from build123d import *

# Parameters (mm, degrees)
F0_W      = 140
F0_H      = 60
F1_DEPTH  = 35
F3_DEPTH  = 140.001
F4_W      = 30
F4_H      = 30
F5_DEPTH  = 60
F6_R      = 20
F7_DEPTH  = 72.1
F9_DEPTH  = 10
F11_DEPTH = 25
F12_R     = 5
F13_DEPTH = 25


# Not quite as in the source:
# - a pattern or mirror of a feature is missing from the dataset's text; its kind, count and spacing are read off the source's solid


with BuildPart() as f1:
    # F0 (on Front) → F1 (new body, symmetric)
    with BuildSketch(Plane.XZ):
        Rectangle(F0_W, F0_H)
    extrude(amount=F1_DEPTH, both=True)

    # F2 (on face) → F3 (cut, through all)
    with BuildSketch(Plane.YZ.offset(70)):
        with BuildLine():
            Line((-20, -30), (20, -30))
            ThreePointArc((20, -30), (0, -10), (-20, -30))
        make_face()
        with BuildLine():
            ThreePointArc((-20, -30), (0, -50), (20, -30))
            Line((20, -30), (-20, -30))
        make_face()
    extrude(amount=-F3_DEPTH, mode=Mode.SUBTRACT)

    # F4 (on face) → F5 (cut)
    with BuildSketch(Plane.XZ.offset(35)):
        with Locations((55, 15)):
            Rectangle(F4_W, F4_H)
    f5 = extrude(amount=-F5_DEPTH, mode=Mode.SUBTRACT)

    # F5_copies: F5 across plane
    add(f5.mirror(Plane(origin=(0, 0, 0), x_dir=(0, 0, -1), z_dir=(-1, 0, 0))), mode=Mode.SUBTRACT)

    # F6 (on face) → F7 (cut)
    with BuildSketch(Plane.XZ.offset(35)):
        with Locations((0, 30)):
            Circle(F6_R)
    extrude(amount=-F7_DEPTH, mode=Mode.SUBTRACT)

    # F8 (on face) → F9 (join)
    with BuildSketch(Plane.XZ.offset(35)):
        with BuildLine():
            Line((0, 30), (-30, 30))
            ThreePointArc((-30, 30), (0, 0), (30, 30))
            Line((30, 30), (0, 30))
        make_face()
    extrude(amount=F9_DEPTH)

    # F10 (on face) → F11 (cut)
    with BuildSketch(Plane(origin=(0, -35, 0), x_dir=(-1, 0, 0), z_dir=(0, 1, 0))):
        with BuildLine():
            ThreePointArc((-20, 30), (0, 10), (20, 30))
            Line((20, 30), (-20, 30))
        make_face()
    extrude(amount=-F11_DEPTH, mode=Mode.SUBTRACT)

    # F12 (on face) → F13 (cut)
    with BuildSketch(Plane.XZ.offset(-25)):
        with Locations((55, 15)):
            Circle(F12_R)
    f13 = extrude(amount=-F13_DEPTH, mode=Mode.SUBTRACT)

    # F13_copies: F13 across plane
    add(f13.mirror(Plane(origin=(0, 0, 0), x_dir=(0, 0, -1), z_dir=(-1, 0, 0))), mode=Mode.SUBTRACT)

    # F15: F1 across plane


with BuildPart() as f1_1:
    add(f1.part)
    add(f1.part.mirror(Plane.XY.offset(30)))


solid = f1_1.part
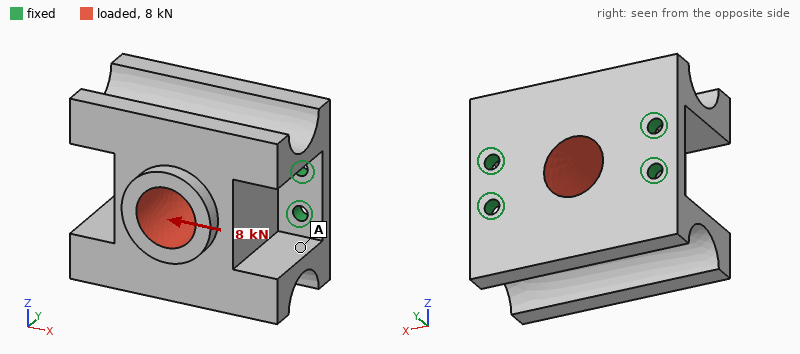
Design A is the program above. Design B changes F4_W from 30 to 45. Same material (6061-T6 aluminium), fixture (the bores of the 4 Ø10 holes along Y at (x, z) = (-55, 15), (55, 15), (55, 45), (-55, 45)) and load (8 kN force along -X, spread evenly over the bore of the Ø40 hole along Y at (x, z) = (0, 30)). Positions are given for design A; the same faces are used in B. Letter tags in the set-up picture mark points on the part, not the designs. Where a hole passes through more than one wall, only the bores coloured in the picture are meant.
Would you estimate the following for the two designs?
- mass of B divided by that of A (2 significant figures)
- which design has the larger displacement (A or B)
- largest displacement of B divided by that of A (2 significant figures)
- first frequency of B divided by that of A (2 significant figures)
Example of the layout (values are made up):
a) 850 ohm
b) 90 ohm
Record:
a) 0.92
b) B
c) 1.3
d) 0.95
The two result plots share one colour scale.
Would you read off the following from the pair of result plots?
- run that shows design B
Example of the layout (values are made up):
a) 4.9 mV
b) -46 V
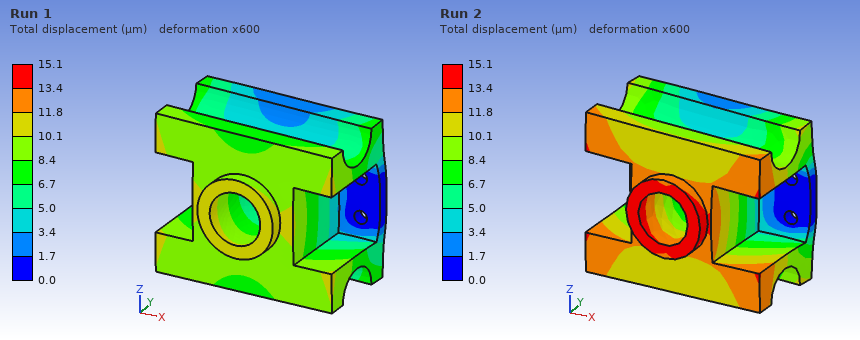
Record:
a) Run 2
